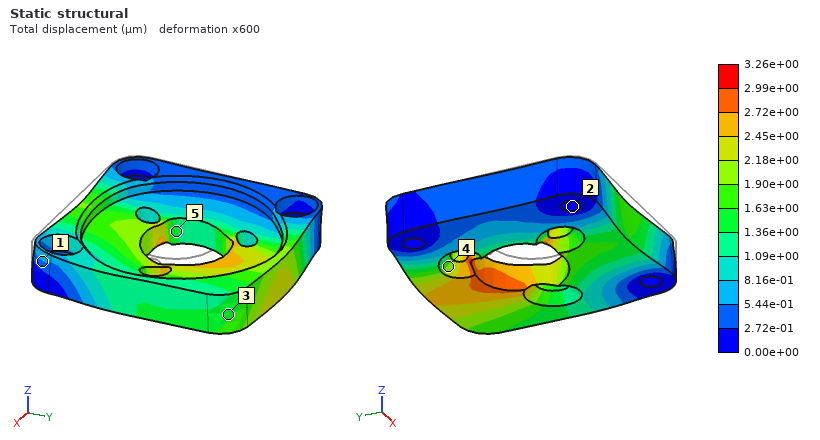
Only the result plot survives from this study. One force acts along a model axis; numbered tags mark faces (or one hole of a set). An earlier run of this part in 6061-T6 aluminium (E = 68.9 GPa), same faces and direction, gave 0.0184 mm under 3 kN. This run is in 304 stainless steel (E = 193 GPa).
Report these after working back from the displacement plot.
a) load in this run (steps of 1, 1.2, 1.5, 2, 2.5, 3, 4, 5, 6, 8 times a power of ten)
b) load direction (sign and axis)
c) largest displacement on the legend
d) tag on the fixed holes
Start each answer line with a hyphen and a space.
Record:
- 1.5 kN
- +Y
- 3.26e+00 µm
- 2
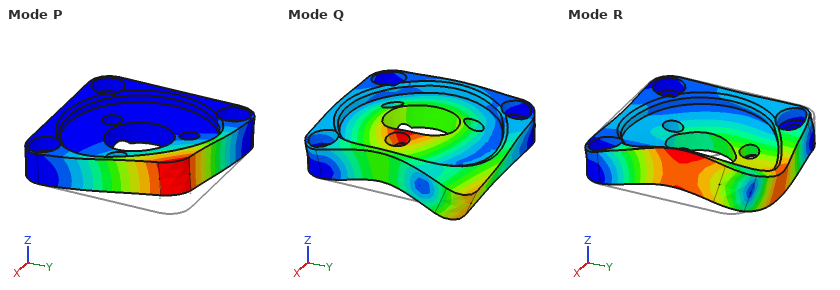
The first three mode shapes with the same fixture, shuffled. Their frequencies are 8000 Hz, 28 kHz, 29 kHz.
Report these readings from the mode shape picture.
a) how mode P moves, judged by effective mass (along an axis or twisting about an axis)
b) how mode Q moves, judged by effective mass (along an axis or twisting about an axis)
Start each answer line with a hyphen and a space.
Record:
- along Z
- along Z
